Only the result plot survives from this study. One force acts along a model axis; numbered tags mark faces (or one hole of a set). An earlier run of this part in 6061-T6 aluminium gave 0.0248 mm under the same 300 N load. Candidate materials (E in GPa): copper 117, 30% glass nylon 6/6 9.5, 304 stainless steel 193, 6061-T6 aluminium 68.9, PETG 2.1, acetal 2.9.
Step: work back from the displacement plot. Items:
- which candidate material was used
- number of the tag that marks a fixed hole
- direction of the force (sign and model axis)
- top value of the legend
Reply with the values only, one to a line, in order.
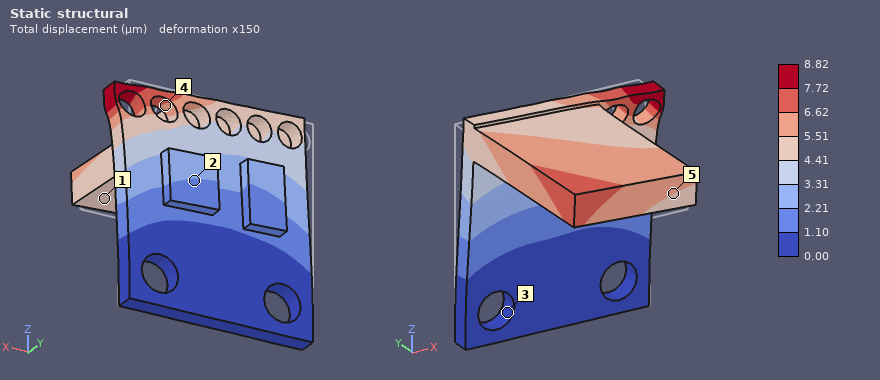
304 stainless steel
3
+X
8.82 µm
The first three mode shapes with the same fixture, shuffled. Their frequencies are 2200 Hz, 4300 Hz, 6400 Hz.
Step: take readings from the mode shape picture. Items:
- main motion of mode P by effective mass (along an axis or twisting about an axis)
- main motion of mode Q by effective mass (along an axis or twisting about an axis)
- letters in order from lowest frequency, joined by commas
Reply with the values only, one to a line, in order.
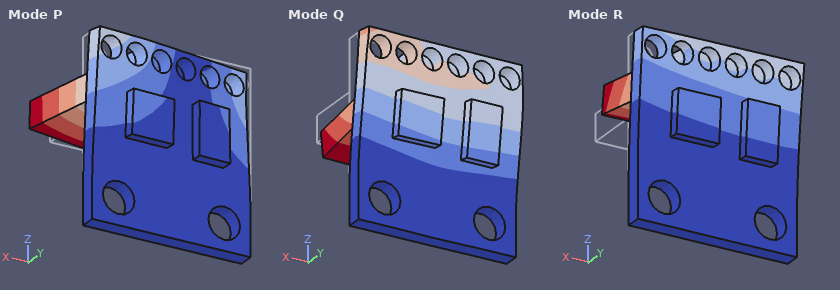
along X
along Y
R, P, Q
